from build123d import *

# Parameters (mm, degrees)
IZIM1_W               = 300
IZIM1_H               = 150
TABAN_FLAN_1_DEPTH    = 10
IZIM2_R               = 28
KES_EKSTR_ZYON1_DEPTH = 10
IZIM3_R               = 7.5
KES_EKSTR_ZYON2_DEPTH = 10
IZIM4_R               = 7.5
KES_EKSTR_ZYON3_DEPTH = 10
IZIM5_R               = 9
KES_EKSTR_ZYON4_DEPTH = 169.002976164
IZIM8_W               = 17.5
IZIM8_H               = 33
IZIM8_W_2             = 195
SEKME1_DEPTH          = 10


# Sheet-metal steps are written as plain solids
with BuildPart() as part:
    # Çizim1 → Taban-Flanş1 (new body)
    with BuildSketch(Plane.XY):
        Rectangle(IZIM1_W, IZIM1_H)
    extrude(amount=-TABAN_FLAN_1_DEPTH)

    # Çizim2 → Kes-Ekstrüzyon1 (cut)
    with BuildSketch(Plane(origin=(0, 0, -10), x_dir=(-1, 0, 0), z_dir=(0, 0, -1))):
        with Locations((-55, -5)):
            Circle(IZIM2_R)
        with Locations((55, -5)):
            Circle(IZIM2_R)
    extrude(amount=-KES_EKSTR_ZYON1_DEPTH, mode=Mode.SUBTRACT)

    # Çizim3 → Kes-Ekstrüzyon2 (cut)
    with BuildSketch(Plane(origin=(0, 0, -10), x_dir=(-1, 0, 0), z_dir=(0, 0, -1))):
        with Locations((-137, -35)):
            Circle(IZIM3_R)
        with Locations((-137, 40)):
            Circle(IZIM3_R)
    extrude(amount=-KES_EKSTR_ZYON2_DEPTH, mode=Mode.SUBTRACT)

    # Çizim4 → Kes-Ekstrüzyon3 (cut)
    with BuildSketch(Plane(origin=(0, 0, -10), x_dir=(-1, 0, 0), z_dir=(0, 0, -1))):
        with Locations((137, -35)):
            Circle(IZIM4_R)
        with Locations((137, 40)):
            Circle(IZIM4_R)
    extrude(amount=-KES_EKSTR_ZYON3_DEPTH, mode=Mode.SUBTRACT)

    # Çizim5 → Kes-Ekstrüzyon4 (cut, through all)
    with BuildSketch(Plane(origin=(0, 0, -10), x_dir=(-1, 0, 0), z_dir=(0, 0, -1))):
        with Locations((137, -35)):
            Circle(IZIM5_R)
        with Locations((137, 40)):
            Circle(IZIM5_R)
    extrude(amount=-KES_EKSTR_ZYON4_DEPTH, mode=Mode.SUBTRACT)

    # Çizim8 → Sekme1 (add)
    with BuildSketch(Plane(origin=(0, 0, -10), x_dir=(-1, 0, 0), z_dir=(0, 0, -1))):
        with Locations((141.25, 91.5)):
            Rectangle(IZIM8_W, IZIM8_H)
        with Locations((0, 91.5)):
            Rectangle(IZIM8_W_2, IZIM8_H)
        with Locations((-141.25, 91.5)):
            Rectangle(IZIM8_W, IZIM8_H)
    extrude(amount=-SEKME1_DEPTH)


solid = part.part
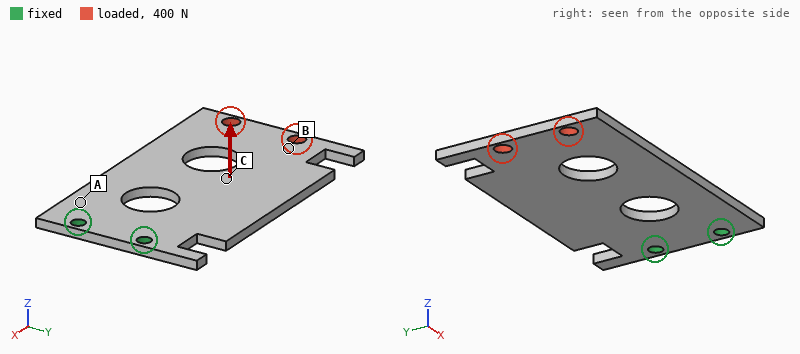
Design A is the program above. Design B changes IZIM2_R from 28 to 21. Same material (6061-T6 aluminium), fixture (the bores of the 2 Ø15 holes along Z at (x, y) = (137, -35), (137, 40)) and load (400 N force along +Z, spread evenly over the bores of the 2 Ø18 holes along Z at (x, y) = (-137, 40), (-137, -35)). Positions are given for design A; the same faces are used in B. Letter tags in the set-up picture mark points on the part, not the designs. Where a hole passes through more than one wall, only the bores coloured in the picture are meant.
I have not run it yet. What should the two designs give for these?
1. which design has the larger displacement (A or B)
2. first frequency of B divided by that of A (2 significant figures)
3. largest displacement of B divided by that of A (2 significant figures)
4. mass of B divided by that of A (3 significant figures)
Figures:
A
1.0
0.92
1.05
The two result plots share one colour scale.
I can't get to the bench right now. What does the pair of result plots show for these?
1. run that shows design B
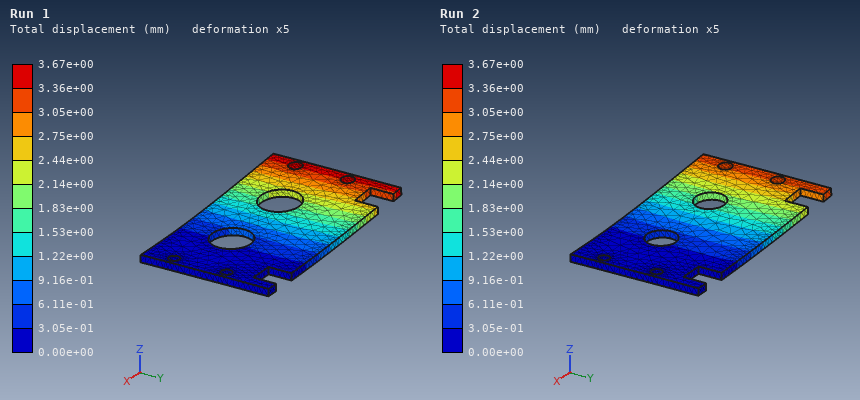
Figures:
Run 2
